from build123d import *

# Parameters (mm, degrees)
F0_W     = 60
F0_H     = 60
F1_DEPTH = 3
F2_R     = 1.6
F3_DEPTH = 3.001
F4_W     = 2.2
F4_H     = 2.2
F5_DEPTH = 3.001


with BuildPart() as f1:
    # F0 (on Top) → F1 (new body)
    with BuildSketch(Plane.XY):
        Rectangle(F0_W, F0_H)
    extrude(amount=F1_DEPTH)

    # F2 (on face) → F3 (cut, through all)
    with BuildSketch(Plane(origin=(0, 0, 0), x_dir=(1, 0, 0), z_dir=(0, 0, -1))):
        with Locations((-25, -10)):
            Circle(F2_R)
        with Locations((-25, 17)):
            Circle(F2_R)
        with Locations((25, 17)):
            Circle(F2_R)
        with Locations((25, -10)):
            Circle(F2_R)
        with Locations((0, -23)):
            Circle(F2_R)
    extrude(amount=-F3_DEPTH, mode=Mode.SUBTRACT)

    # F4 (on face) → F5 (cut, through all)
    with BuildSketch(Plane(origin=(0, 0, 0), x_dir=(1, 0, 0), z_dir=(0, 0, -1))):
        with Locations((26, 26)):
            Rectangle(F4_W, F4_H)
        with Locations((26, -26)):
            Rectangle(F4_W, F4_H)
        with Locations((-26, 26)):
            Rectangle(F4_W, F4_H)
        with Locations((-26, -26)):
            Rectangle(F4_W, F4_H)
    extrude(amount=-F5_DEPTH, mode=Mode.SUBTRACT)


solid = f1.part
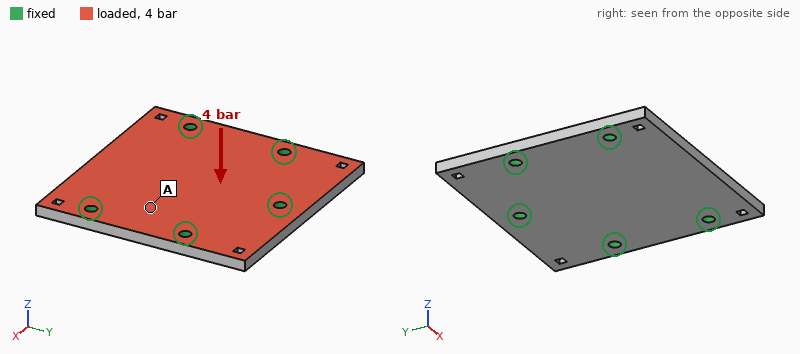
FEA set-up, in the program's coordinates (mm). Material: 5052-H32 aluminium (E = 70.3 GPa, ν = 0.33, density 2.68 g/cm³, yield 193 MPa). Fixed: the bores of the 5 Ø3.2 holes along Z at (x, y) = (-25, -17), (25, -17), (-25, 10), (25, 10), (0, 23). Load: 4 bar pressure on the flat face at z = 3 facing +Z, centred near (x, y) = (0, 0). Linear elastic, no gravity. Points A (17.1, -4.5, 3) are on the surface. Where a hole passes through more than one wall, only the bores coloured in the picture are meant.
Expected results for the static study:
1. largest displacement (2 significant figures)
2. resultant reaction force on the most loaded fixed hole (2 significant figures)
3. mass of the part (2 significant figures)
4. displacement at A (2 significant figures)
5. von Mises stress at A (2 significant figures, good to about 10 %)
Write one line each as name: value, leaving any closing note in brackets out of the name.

largest displacement: 67 µm
resultant reaction force on the most loaded fixed hole: 320 N
mass of the part: 28 g
displacement at A: 16 µm
von Mises stress at A: 12 MPa
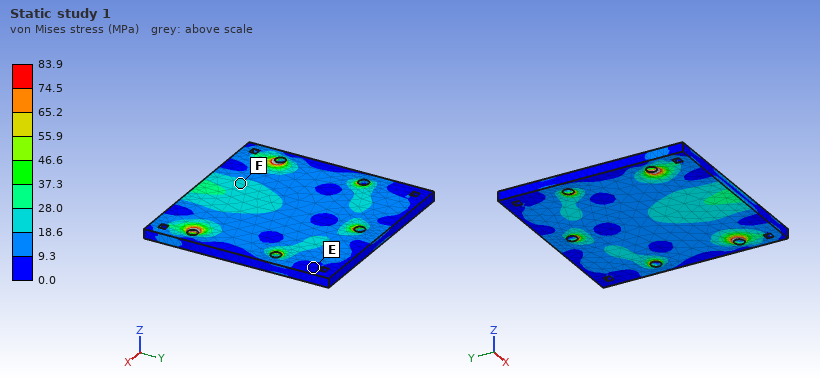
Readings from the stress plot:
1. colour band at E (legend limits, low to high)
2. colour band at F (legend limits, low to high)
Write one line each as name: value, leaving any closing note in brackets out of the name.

colour band at E: 0.0 to 9.3 MPa
colour band at F: 18.6 to 28.0 MPa
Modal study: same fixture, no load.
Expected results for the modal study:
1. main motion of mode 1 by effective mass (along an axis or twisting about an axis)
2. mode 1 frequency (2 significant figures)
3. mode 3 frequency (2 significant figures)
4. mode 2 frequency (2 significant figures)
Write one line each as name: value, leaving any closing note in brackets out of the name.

main motion of mode 1 by effective mass: along Z
mode 1 frequency: 5700 Hz
mode 3 frequency: 8700 Hz
mode 2 frequency: 8300 Hz
